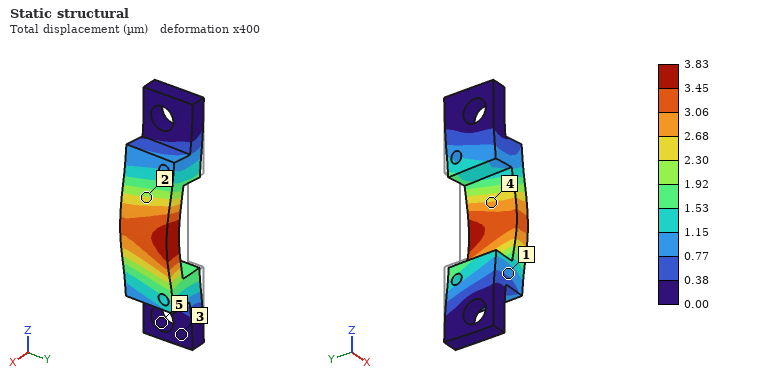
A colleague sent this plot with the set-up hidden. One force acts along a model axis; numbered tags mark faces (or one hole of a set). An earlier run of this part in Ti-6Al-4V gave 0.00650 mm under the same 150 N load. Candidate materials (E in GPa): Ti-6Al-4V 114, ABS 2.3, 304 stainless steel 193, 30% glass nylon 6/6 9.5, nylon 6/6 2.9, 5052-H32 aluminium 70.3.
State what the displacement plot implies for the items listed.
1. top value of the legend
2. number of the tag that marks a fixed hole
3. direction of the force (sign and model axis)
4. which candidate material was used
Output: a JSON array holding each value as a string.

["3.83 µm", "5", "+X", "304 stainless steel"]
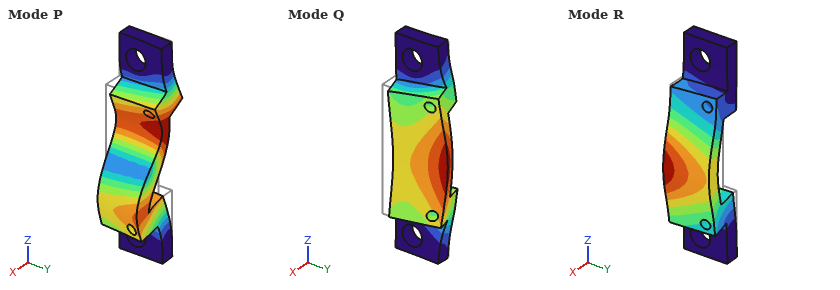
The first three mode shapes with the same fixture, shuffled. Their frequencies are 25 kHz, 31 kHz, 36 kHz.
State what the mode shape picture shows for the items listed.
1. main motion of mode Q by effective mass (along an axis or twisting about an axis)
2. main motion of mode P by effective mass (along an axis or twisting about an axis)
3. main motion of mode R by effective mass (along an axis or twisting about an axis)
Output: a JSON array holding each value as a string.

["along Y", "along Z", "along X"]
